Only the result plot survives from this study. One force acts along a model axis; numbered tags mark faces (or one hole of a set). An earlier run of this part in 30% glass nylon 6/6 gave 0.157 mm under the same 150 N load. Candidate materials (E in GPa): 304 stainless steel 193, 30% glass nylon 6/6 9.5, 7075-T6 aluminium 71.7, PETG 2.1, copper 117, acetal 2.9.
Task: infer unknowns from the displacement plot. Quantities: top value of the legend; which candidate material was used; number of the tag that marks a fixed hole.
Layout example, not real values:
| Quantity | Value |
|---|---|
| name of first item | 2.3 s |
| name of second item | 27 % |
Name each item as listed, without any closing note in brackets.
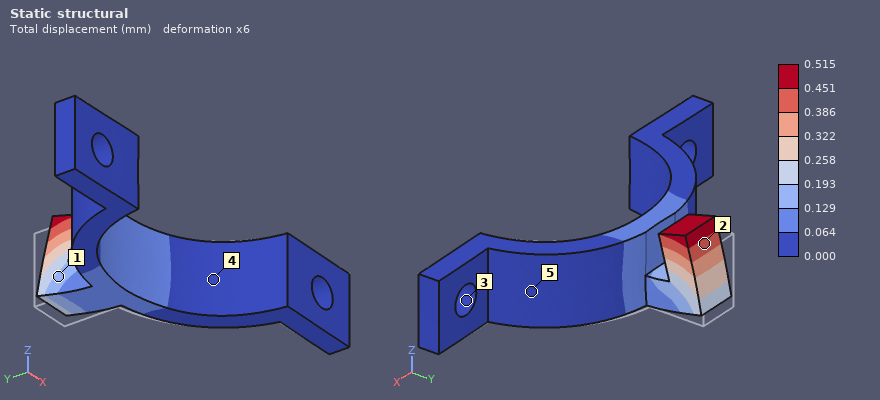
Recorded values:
| Quantity | Value |
|---|---|
| top value of the legend | 0.515 mm |
| which candidate material was used | acetal |
| number of the tag that marks a fixed hole | 3 |
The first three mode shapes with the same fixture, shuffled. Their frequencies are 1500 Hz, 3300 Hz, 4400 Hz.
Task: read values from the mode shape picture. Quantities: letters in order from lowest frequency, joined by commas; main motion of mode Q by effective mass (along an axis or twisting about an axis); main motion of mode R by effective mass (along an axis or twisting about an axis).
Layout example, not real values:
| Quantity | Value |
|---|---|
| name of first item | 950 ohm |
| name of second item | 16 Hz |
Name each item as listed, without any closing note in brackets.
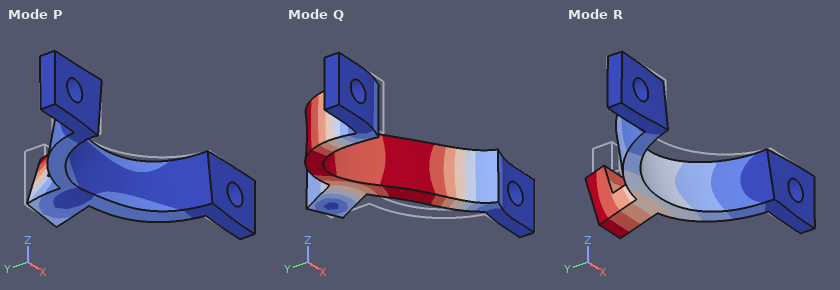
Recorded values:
| Quantity | Value |
|---|---|
| letters in order from lowest frequency, joined by commas | R, Q, P |
| main motion of mode Q by effective mass | along X |
| main motion of mode R by effective mass | along Z |
